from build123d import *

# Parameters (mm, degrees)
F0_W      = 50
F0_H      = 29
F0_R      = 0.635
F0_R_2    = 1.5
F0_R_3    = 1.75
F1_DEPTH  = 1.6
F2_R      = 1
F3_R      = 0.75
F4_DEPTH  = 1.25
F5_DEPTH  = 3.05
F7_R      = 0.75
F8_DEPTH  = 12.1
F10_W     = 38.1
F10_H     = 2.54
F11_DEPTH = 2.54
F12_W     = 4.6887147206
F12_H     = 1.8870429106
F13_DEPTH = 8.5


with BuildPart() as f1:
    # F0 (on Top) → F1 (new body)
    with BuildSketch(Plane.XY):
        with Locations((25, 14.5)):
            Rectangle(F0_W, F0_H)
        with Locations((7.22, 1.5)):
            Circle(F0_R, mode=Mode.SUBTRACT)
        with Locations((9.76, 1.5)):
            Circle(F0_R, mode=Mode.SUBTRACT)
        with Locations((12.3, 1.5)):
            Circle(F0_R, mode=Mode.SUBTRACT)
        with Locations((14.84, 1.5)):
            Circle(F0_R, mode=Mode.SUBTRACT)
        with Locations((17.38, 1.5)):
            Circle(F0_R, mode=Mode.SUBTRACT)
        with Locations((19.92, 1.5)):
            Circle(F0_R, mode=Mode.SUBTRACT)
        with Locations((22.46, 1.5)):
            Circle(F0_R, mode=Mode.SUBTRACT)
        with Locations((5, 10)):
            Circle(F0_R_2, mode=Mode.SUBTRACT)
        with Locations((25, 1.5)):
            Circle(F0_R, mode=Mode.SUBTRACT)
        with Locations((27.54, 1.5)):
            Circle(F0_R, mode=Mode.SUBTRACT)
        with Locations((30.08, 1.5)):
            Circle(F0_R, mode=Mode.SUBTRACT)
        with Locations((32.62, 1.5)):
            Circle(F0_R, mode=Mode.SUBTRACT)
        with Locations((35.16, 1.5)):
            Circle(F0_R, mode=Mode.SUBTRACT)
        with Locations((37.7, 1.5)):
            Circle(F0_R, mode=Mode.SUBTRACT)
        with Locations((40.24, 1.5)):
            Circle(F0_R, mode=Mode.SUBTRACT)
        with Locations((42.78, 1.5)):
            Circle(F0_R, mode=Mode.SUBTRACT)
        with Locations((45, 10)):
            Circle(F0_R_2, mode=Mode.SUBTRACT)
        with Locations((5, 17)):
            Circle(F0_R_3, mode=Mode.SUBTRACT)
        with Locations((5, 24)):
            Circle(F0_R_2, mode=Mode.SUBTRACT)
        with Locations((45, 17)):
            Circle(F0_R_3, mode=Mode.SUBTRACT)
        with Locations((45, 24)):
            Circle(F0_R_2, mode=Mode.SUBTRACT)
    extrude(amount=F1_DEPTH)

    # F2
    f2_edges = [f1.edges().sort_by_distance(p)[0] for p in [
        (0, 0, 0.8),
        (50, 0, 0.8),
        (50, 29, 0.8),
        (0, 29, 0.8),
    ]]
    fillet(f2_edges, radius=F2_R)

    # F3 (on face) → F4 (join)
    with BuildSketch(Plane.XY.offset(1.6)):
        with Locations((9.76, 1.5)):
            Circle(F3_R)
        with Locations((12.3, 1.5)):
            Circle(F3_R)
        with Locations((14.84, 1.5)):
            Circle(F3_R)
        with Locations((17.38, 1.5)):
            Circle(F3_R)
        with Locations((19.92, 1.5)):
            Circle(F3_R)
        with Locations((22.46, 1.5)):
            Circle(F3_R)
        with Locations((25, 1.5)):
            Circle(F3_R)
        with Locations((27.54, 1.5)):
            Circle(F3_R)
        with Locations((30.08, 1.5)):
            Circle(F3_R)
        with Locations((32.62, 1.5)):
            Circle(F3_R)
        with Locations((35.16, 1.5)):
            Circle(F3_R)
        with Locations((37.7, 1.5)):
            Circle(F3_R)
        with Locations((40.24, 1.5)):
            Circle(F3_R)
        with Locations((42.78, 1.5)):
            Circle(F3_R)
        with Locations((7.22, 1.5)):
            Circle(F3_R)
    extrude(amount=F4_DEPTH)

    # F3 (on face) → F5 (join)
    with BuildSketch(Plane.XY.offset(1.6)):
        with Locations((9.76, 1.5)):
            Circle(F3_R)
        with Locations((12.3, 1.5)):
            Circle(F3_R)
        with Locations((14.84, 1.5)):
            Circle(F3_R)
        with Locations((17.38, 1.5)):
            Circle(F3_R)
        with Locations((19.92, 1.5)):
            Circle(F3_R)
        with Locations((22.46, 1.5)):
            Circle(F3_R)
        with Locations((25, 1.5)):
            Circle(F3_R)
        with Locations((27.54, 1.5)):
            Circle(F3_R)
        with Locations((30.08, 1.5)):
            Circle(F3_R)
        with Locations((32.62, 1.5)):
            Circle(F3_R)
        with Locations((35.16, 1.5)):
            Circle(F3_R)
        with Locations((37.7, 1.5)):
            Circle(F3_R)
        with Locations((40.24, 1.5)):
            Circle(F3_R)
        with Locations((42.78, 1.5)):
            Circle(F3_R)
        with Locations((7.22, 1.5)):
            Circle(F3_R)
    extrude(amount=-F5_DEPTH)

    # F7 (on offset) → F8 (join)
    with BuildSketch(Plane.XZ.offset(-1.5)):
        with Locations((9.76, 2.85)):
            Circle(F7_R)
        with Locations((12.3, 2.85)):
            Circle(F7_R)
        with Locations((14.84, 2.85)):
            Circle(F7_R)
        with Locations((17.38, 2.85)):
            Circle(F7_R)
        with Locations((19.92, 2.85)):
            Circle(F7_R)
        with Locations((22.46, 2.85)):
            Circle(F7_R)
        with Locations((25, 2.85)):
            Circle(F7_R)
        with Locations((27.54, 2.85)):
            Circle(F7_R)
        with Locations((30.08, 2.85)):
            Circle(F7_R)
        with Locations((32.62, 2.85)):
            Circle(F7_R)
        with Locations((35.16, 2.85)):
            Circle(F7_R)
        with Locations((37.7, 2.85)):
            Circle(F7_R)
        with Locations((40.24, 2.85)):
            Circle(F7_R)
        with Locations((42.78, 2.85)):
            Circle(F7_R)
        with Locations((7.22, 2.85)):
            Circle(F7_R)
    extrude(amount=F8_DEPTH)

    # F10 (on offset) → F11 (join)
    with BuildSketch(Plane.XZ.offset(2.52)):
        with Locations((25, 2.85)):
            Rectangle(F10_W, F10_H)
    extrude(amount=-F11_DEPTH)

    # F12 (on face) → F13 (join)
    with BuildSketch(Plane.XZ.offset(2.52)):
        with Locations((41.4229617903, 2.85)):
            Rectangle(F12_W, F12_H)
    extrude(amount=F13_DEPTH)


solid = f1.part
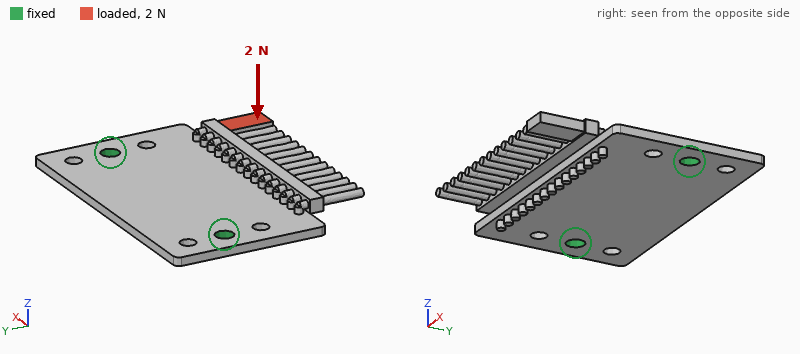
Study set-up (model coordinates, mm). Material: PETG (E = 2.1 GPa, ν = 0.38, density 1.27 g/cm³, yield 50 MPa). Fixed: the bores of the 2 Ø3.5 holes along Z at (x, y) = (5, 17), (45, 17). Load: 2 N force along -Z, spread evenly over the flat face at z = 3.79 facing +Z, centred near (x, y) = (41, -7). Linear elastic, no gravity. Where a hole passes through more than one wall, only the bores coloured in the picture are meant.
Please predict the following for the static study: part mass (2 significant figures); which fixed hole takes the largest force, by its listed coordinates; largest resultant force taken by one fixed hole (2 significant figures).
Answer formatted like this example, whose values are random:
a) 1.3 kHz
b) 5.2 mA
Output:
a) 3.6 g
b) (45, 17)
c) 1.9 N
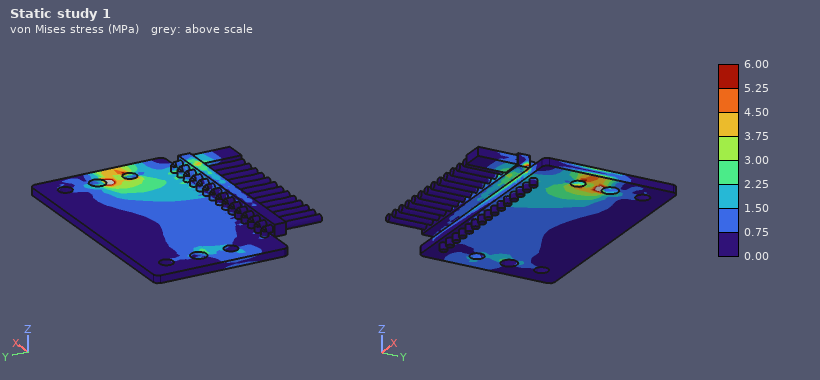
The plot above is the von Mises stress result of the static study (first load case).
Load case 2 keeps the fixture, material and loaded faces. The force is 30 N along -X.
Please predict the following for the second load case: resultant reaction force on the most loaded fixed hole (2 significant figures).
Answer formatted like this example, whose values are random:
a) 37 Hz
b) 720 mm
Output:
a) 24 N
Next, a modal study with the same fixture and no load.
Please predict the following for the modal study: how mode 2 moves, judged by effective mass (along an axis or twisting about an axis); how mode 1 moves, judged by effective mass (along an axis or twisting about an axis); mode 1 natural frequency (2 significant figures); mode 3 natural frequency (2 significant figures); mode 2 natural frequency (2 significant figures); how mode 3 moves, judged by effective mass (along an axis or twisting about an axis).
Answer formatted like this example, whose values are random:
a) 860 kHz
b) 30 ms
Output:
a) twisting about Y
b) along Z
c) 470 Hz
d) 1300 Hz
e) 940 Hz
f) along Z
